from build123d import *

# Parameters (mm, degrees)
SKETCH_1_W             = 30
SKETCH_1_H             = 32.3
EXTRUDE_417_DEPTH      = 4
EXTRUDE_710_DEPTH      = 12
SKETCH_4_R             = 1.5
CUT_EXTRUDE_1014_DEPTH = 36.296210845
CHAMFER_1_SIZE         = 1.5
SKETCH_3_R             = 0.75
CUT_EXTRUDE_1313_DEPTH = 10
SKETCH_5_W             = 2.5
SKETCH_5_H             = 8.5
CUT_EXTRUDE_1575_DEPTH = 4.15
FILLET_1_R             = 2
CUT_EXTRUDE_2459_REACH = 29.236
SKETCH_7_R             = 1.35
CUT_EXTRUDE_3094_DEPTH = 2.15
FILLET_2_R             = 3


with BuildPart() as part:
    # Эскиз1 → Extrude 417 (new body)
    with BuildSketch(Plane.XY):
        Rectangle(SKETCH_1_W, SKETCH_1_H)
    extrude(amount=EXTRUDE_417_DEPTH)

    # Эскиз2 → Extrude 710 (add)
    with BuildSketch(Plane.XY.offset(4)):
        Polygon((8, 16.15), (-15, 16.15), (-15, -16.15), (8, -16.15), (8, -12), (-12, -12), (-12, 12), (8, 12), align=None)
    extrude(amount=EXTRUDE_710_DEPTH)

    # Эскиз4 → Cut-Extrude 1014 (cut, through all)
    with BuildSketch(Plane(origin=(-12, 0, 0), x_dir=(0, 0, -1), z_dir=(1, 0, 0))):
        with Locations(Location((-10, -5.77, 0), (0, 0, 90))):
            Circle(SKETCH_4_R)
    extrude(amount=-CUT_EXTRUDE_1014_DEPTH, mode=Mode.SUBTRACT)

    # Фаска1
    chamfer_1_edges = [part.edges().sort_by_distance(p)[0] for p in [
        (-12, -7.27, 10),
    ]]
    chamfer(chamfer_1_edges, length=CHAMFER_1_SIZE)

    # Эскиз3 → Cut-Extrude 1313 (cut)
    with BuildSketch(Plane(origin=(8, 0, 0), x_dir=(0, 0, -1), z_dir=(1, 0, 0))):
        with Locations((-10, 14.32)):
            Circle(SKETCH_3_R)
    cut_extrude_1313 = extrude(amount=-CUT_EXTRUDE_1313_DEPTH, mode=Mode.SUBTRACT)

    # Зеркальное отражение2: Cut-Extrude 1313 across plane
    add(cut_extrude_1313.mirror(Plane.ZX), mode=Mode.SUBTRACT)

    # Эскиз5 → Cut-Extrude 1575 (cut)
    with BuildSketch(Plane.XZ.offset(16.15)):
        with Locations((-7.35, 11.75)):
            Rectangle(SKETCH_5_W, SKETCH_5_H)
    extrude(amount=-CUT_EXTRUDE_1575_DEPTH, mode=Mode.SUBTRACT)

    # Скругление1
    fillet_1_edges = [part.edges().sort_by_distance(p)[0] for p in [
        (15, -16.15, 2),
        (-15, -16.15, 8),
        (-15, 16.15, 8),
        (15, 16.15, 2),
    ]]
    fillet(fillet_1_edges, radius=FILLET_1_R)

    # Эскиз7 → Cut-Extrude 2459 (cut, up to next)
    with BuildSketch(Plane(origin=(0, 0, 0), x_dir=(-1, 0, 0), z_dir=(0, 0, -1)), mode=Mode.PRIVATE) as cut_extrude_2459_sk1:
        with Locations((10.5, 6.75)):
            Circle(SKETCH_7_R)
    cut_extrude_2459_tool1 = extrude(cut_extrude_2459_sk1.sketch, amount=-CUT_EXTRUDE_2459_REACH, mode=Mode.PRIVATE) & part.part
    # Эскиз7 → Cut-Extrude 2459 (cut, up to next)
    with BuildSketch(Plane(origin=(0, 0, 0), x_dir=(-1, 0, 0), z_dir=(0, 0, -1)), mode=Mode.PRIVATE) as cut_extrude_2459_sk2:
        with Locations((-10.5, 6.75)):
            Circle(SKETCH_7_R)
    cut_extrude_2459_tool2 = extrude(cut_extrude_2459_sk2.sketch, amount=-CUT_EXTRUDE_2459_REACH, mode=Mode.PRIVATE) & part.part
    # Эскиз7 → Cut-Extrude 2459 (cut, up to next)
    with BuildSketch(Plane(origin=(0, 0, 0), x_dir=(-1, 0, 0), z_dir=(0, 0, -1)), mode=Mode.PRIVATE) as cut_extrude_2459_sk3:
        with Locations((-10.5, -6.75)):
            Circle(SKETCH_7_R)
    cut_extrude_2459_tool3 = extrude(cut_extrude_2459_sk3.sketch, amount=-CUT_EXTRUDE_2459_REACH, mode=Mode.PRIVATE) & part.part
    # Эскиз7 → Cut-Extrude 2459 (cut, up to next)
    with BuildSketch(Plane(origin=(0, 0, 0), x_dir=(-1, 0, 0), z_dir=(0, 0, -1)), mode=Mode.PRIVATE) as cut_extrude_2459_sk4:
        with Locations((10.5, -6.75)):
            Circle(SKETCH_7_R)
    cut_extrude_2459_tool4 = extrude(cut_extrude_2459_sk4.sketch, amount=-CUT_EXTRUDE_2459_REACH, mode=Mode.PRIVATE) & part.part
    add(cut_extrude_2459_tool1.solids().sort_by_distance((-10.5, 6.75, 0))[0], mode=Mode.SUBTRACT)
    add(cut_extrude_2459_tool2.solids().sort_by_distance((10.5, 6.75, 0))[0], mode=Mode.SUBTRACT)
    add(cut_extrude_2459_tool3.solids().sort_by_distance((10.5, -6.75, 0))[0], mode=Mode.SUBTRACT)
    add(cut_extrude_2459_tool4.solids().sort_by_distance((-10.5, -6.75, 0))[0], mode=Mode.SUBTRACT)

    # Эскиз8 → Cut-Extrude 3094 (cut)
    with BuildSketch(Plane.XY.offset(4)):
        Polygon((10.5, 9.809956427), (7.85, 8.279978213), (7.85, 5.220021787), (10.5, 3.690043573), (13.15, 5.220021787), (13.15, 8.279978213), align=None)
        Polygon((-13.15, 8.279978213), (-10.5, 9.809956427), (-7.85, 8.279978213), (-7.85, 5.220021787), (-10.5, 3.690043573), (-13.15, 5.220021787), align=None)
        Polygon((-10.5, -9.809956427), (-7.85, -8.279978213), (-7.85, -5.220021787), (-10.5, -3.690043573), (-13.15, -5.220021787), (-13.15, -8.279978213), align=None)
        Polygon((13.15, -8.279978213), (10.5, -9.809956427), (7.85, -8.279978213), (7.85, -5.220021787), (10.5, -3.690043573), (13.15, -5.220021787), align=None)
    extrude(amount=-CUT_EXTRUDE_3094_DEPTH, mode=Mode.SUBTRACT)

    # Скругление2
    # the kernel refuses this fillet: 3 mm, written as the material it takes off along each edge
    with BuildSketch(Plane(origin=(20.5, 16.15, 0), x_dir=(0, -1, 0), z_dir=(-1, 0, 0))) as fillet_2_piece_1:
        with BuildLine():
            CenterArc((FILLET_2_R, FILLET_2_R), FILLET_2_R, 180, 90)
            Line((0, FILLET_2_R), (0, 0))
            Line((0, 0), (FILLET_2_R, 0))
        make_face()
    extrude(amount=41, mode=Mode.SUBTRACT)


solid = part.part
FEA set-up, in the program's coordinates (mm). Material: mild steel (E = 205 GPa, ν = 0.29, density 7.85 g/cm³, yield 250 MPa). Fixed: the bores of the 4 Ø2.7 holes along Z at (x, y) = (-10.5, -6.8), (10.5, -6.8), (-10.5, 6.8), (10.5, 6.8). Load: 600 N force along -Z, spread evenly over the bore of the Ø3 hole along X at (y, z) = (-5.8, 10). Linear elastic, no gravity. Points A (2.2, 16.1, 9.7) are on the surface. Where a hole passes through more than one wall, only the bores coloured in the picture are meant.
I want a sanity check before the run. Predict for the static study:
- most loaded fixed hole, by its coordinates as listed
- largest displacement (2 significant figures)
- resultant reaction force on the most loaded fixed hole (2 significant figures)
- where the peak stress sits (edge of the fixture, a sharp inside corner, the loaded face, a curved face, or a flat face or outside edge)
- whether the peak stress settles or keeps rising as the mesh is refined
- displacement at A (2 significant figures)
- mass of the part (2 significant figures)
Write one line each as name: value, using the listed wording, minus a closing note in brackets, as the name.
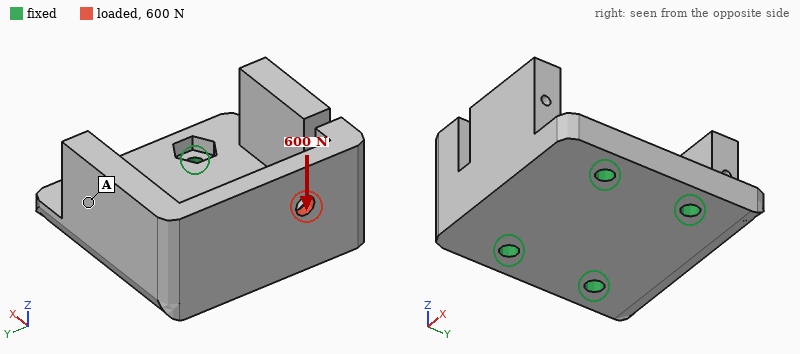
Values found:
most loaded fixed hole, by its coordinates as listed: (-10.5, -6.8)
largest displacement: 5.5 µm
resultant reaction force on the most loaded fixed hole: 570 N
where the peak stress sits: edge of the fixture
whether the peak stress settles or keeps rising as the mesh is refined: keeps rising
displacement at A: 1.3 µm
mass of the part: 51 g
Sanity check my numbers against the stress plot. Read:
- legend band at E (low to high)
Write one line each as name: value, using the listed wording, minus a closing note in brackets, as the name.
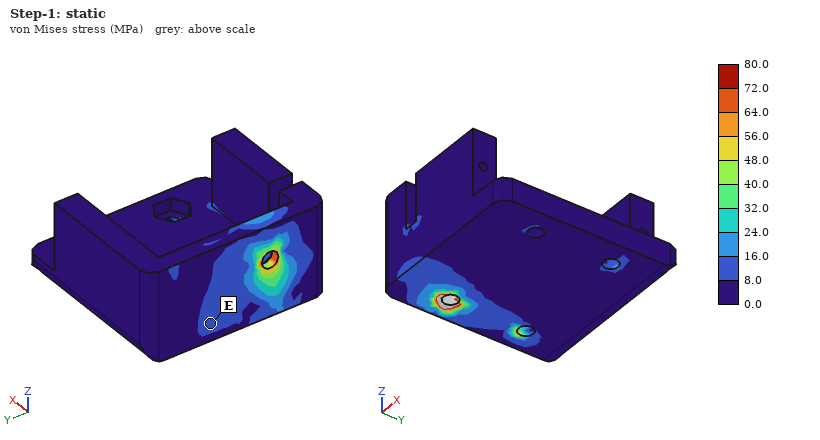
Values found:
legend band at E: 8.0 to 16.0 MPa
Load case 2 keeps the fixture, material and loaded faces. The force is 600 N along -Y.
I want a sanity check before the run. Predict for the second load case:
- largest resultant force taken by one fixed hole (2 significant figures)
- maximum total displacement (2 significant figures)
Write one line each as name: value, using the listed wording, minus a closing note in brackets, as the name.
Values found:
largest resultant force taken by one fixed hole: 460 N
maximum total displacement: 5.2 µm
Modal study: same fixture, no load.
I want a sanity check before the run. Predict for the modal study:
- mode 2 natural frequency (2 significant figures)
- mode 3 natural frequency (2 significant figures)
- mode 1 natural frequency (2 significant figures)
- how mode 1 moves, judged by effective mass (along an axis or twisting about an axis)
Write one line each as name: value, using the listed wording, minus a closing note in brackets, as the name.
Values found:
mode 2 natural frequency: 12 kHz
mode 3 natural frequency: 15 kHz
mode 1 natural frequency: 10 kHz
how mode 1 moves, judged by effective mass: along Y
